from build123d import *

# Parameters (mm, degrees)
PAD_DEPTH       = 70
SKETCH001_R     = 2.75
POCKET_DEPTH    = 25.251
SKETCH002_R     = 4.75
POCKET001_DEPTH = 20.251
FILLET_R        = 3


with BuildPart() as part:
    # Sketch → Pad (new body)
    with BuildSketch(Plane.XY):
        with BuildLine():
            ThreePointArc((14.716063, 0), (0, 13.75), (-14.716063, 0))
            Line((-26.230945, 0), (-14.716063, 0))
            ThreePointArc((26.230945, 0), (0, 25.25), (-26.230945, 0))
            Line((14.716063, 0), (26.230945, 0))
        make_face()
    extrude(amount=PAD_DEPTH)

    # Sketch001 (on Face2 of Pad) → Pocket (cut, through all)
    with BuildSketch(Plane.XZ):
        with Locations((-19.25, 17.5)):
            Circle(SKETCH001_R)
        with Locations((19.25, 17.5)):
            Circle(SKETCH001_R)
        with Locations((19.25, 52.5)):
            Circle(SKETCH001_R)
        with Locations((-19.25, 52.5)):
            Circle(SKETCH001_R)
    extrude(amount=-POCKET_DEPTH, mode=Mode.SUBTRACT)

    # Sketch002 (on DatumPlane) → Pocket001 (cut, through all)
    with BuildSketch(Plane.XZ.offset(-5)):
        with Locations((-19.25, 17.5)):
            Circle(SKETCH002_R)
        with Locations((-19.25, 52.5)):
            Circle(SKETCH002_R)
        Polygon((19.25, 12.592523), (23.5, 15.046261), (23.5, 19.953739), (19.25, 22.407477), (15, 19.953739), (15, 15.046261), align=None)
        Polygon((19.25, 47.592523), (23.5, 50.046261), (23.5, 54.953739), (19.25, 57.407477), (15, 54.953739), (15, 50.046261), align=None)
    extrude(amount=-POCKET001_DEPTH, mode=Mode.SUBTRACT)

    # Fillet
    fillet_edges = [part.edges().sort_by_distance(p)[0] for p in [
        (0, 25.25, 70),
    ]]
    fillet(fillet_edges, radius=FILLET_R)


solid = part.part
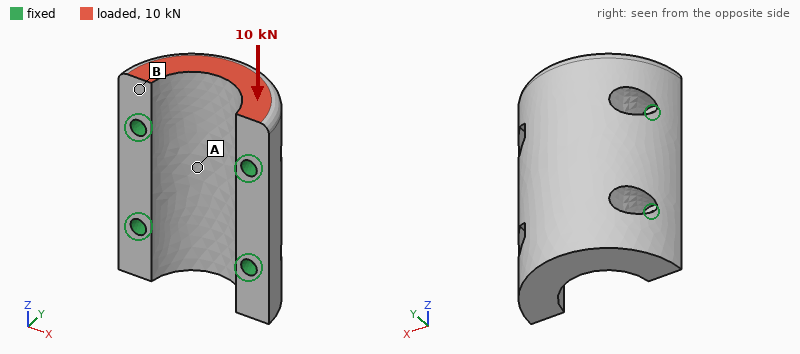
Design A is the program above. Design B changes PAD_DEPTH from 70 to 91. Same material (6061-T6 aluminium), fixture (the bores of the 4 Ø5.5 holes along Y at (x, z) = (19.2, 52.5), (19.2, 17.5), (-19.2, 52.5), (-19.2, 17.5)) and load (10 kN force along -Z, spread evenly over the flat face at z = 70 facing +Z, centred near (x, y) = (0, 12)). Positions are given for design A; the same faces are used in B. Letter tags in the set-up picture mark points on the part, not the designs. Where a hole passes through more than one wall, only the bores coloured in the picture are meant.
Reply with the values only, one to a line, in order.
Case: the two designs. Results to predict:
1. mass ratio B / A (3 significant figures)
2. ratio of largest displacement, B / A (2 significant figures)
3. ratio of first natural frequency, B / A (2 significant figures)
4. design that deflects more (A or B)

1.32
1.5
0.53
B
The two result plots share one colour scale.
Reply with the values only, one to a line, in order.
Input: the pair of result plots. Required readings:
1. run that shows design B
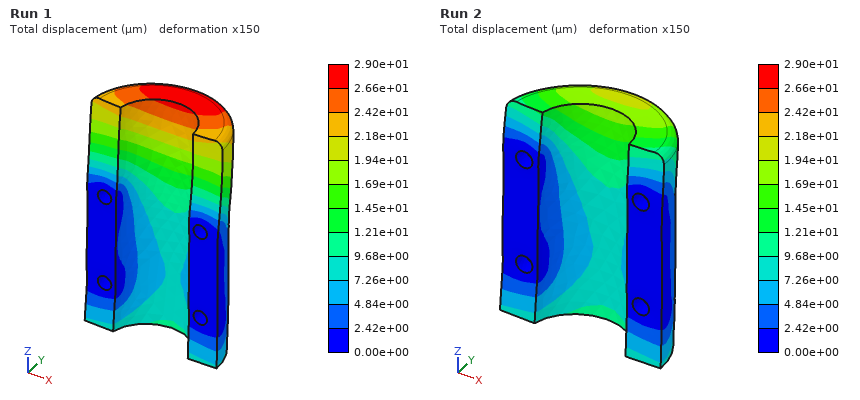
Run 1
